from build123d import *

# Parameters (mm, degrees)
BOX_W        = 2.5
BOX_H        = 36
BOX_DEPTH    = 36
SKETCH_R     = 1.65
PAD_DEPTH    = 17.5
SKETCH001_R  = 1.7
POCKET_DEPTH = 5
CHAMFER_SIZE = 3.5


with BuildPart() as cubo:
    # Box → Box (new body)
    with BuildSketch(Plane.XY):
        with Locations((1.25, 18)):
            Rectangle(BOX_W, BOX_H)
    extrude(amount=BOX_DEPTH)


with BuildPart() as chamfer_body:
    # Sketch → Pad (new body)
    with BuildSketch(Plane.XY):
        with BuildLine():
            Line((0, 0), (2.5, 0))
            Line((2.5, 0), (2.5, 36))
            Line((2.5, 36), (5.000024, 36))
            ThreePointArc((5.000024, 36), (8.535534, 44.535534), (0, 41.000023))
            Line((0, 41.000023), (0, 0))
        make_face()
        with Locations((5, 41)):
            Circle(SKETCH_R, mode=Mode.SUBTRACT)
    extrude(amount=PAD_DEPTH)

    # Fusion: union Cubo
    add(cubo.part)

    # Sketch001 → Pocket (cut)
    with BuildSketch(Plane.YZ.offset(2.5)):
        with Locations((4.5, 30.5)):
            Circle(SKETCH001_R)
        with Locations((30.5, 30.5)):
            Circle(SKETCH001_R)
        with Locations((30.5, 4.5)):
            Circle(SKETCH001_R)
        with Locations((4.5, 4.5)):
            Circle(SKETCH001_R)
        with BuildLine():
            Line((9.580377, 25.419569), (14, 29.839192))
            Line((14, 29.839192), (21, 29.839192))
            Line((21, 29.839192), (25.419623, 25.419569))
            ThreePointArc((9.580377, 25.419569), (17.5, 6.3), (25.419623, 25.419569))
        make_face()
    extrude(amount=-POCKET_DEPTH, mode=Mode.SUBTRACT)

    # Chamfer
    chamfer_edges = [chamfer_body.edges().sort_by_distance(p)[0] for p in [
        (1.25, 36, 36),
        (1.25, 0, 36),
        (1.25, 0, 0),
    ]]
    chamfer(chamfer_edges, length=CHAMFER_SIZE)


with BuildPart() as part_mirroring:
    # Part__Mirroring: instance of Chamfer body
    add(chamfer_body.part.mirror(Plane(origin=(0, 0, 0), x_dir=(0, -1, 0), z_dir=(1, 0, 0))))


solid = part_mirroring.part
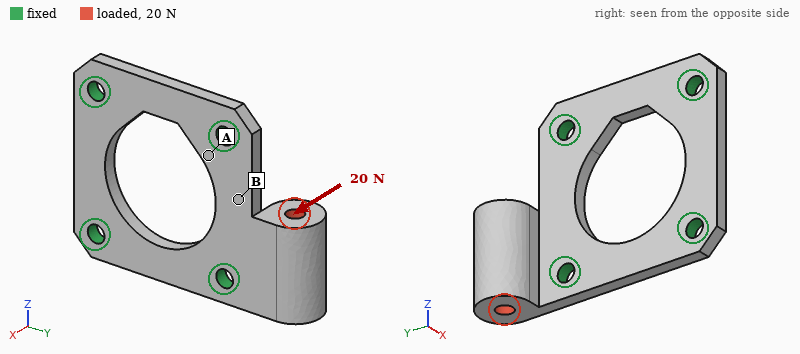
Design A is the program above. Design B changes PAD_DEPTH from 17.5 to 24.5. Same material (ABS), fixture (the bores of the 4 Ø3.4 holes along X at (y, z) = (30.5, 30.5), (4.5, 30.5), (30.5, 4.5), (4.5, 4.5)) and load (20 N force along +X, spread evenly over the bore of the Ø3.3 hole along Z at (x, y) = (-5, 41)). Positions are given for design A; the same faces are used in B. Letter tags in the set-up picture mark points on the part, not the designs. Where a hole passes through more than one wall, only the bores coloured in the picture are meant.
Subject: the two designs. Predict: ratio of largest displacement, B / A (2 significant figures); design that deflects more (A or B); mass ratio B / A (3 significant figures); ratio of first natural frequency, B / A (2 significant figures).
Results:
0.77
A
1.16
0.95
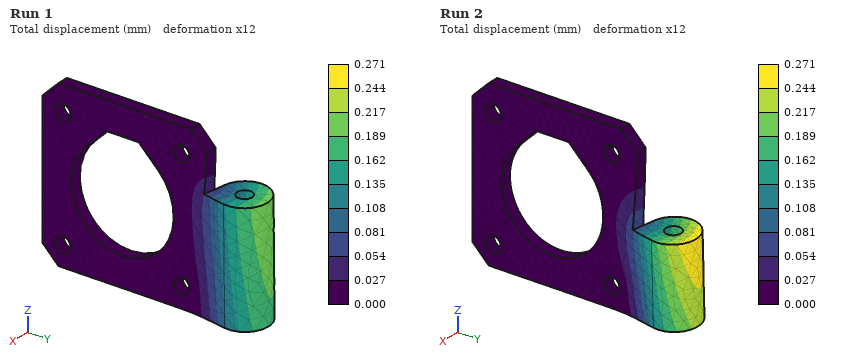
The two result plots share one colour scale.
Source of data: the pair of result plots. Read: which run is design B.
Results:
Run 1
